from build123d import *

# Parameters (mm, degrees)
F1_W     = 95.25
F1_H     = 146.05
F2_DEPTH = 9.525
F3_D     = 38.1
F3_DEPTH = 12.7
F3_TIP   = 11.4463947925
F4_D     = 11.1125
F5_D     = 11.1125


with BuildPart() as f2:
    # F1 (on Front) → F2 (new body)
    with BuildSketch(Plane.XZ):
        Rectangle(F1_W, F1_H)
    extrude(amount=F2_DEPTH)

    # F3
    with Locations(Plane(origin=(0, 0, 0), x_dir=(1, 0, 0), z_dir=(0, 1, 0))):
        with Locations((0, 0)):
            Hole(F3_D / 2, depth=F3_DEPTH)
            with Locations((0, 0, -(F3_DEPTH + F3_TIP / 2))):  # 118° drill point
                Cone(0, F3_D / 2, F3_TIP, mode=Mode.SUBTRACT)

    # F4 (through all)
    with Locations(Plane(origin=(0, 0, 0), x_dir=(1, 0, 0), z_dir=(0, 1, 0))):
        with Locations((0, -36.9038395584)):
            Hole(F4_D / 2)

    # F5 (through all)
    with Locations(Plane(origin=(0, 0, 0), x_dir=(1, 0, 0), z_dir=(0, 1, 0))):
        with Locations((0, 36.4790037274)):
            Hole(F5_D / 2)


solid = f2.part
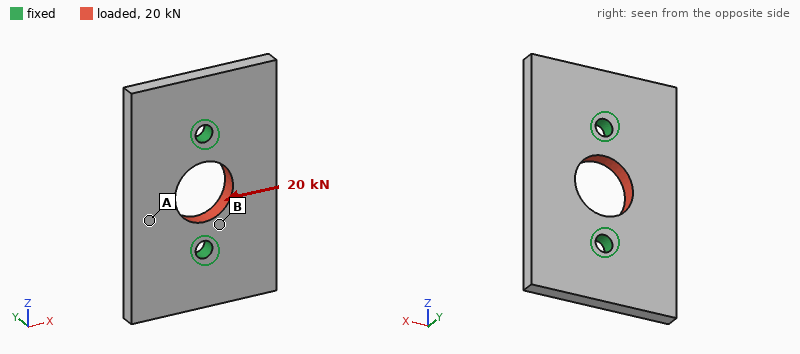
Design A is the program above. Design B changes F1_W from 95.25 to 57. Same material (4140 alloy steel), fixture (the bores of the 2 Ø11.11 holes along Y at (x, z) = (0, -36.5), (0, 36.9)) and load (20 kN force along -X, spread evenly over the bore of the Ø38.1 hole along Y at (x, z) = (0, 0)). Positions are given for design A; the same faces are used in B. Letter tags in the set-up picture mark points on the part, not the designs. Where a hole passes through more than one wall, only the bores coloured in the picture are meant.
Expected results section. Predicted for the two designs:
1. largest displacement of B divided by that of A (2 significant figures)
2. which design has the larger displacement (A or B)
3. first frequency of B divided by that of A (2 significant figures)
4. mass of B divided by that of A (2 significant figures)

2.1
B
2.0
0.56
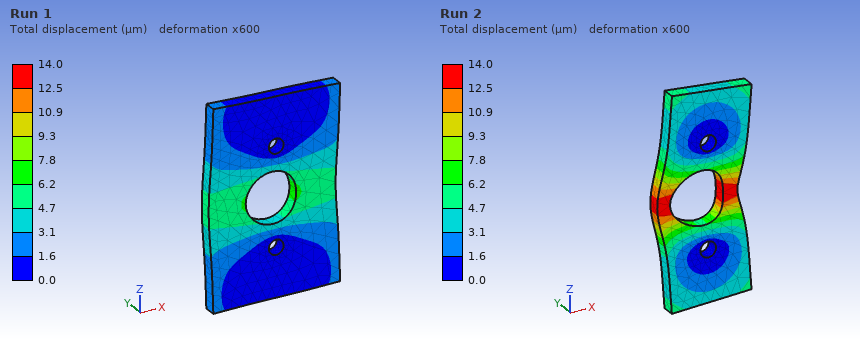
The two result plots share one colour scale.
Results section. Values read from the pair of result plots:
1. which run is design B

Run 2
